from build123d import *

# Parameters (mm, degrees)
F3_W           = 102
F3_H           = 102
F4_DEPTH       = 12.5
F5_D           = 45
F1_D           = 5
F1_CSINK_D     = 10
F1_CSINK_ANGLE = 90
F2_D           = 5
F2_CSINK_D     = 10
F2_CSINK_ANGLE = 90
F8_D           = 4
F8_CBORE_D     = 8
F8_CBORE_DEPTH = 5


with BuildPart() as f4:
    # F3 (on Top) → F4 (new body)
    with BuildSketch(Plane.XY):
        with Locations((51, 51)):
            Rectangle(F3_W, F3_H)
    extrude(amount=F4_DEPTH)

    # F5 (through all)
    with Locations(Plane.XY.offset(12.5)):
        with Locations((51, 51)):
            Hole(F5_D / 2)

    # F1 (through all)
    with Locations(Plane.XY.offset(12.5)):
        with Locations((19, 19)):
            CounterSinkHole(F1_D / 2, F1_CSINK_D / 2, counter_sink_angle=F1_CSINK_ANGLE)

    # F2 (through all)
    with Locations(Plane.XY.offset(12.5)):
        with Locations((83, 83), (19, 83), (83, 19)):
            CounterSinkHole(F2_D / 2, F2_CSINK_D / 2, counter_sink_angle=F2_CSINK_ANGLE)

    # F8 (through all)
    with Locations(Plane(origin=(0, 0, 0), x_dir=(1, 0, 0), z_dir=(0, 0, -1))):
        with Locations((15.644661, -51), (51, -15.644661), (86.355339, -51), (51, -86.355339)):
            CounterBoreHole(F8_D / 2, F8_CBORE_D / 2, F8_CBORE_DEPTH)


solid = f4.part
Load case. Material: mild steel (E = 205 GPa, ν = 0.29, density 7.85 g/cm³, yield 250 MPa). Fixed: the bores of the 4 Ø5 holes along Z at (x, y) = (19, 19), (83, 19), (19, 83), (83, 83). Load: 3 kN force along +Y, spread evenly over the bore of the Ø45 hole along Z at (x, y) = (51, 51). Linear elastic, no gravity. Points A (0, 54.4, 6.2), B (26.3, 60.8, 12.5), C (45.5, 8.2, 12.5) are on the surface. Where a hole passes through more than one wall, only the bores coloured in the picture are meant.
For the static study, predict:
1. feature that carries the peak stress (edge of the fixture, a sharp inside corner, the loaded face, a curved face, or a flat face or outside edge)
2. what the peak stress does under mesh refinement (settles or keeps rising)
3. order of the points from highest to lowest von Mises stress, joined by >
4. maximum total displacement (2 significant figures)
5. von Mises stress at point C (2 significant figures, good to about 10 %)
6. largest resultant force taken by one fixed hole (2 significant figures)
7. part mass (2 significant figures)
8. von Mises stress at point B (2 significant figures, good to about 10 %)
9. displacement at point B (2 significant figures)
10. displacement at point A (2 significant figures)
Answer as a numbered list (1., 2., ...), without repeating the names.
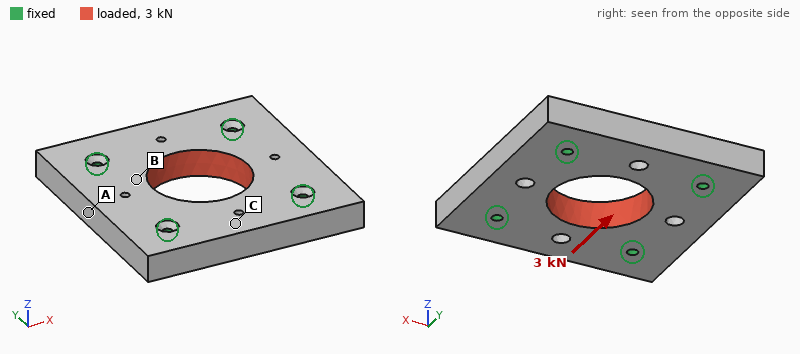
1. edge of the fixture
2. keeps rising
3. B > C > A
4. 0.65 µm
5. 1.4 MPa
6. 760 N
7. 840 g
8. 2.6 MPa
9. 0.30 µm
10. 0.11 µm
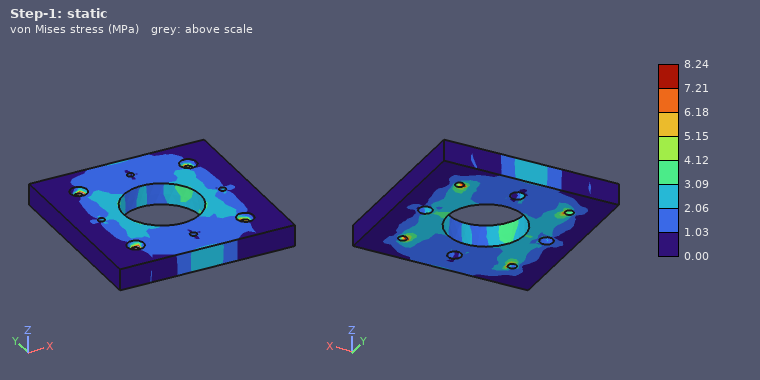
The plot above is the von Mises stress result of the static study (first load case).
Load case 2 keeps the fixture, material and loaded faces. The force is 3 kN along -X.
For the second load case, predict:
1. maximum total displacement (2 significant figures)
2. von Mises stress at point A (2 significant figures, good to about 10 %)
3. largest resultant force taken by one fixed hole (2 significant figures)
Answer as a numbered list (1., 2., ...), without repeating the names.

1. 0.65 µm
2. 2.4 MPa
3. 760 N
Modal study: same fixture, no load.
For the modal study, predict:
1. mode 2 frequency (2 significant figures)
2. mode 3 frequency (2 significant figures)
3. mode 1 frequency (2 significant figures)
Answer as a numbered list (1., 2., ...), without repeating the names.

1. 10 kHz
2. 10 kHz
3. 8800 Hz
